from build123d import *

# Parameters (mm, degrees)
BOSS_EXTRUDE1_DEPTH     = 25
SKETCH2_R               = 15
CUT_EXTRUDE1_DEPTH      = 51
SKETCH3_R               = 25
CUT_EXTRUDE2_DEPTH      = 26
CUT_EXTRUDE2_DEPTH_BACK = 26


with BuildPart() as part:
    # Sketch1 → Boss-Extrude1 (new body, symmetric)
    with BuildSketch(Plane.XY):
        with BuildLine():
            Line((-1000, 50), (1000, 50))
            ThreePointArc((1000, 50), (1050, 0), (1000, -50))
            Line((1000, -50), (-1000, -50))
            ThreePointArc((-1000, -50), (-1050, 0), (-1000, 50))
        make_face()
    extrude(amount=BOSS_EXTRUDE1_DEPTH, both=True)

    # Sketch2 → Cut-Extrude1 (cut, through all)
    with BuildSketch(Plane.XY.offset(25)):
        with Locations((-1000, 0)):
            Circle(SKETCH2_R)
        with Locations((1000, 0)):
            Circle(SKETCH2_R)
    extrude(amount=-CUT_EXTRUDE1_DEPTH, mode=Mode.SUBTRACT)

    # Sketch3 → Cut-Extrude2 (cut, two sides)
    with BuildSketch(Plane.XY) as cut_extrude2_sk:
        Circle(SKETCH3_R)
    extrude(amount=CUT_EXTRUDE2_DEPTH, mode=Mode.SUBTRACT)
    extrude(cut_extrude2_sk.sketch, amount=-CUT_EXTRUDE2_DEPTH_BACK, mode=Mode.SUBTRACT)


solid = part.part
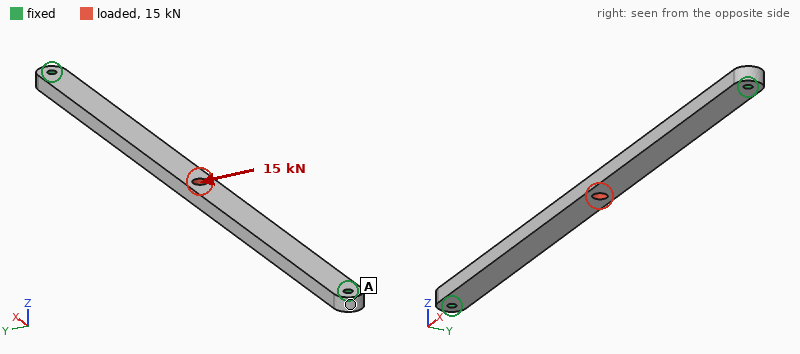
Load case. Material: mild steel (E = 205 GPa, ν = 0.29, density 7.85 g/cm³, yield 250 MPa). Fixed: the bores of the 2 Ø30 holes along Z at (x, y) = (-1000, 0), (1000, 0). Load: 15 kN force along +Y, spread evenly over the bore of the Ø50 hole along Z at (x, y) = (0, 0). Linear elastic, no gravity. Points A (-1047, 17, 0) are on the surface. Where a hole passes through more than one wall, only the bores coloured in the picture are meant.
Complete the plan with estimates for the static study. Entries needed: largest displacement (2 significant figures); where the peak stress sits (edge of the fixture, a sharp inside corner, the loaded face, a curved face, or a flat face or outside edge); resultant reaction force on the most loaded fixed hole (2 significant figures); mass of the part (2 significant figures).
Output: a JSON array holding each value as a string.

["0.88 mm", "edge of the fixture", "7.5 kN", "80 kg"]
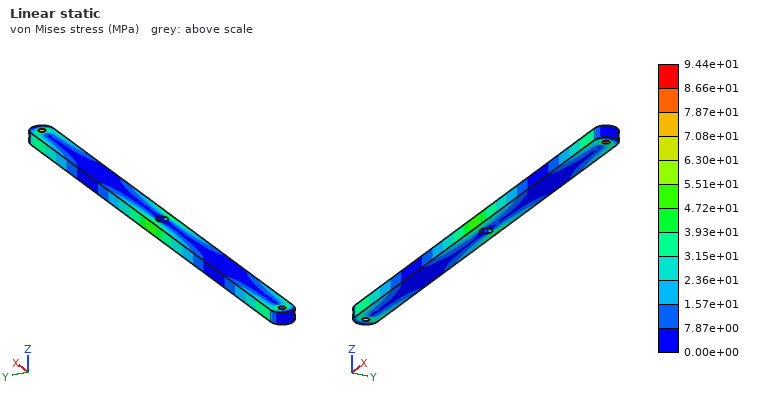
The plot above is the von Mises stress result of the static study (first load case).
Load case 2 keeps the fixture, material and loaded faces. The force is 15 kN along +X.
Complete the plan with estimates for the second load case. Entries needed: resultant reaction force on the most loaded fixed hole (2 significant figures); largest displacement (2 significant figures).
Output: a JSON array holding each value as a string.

["7.5 kN", "7.4 µm"]
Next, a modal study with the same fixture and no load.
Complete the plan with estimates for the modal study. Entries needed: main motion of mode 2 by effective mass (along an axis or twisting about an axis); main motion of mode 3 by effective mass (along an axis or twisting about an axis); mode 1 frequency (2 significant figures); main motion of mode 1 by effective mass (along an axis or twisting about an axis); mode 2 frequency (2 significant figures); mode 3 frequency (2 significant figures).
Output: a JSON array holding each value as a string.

["along Y", "twisting about Y", "65 Hz", "along Z", "120 Hz", "180 Hz"]
